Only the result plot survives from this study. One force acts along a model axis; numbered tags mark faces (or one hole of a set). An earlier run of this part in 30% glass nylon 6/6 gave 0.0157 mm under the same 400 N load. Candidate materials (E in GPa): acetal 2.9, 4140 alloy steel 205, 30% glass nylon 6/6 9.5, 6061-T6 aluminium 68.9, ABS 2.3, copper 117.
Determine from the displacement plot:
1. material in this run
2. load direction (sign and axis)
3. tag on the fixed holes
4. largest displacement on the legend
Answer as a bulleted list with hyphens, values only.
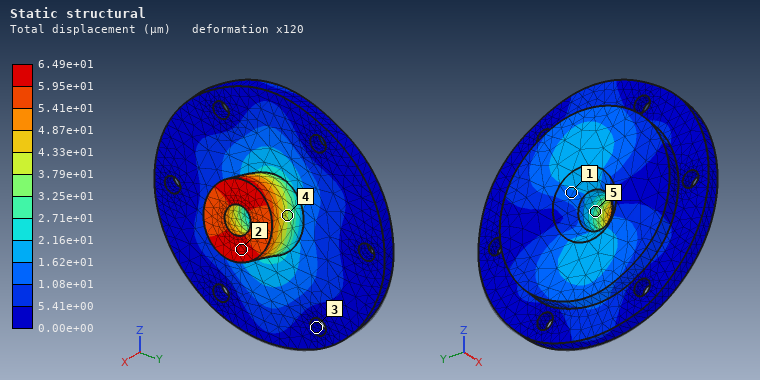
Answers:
- ABS
- +Z
- 3
- 6.49e+01 µm
